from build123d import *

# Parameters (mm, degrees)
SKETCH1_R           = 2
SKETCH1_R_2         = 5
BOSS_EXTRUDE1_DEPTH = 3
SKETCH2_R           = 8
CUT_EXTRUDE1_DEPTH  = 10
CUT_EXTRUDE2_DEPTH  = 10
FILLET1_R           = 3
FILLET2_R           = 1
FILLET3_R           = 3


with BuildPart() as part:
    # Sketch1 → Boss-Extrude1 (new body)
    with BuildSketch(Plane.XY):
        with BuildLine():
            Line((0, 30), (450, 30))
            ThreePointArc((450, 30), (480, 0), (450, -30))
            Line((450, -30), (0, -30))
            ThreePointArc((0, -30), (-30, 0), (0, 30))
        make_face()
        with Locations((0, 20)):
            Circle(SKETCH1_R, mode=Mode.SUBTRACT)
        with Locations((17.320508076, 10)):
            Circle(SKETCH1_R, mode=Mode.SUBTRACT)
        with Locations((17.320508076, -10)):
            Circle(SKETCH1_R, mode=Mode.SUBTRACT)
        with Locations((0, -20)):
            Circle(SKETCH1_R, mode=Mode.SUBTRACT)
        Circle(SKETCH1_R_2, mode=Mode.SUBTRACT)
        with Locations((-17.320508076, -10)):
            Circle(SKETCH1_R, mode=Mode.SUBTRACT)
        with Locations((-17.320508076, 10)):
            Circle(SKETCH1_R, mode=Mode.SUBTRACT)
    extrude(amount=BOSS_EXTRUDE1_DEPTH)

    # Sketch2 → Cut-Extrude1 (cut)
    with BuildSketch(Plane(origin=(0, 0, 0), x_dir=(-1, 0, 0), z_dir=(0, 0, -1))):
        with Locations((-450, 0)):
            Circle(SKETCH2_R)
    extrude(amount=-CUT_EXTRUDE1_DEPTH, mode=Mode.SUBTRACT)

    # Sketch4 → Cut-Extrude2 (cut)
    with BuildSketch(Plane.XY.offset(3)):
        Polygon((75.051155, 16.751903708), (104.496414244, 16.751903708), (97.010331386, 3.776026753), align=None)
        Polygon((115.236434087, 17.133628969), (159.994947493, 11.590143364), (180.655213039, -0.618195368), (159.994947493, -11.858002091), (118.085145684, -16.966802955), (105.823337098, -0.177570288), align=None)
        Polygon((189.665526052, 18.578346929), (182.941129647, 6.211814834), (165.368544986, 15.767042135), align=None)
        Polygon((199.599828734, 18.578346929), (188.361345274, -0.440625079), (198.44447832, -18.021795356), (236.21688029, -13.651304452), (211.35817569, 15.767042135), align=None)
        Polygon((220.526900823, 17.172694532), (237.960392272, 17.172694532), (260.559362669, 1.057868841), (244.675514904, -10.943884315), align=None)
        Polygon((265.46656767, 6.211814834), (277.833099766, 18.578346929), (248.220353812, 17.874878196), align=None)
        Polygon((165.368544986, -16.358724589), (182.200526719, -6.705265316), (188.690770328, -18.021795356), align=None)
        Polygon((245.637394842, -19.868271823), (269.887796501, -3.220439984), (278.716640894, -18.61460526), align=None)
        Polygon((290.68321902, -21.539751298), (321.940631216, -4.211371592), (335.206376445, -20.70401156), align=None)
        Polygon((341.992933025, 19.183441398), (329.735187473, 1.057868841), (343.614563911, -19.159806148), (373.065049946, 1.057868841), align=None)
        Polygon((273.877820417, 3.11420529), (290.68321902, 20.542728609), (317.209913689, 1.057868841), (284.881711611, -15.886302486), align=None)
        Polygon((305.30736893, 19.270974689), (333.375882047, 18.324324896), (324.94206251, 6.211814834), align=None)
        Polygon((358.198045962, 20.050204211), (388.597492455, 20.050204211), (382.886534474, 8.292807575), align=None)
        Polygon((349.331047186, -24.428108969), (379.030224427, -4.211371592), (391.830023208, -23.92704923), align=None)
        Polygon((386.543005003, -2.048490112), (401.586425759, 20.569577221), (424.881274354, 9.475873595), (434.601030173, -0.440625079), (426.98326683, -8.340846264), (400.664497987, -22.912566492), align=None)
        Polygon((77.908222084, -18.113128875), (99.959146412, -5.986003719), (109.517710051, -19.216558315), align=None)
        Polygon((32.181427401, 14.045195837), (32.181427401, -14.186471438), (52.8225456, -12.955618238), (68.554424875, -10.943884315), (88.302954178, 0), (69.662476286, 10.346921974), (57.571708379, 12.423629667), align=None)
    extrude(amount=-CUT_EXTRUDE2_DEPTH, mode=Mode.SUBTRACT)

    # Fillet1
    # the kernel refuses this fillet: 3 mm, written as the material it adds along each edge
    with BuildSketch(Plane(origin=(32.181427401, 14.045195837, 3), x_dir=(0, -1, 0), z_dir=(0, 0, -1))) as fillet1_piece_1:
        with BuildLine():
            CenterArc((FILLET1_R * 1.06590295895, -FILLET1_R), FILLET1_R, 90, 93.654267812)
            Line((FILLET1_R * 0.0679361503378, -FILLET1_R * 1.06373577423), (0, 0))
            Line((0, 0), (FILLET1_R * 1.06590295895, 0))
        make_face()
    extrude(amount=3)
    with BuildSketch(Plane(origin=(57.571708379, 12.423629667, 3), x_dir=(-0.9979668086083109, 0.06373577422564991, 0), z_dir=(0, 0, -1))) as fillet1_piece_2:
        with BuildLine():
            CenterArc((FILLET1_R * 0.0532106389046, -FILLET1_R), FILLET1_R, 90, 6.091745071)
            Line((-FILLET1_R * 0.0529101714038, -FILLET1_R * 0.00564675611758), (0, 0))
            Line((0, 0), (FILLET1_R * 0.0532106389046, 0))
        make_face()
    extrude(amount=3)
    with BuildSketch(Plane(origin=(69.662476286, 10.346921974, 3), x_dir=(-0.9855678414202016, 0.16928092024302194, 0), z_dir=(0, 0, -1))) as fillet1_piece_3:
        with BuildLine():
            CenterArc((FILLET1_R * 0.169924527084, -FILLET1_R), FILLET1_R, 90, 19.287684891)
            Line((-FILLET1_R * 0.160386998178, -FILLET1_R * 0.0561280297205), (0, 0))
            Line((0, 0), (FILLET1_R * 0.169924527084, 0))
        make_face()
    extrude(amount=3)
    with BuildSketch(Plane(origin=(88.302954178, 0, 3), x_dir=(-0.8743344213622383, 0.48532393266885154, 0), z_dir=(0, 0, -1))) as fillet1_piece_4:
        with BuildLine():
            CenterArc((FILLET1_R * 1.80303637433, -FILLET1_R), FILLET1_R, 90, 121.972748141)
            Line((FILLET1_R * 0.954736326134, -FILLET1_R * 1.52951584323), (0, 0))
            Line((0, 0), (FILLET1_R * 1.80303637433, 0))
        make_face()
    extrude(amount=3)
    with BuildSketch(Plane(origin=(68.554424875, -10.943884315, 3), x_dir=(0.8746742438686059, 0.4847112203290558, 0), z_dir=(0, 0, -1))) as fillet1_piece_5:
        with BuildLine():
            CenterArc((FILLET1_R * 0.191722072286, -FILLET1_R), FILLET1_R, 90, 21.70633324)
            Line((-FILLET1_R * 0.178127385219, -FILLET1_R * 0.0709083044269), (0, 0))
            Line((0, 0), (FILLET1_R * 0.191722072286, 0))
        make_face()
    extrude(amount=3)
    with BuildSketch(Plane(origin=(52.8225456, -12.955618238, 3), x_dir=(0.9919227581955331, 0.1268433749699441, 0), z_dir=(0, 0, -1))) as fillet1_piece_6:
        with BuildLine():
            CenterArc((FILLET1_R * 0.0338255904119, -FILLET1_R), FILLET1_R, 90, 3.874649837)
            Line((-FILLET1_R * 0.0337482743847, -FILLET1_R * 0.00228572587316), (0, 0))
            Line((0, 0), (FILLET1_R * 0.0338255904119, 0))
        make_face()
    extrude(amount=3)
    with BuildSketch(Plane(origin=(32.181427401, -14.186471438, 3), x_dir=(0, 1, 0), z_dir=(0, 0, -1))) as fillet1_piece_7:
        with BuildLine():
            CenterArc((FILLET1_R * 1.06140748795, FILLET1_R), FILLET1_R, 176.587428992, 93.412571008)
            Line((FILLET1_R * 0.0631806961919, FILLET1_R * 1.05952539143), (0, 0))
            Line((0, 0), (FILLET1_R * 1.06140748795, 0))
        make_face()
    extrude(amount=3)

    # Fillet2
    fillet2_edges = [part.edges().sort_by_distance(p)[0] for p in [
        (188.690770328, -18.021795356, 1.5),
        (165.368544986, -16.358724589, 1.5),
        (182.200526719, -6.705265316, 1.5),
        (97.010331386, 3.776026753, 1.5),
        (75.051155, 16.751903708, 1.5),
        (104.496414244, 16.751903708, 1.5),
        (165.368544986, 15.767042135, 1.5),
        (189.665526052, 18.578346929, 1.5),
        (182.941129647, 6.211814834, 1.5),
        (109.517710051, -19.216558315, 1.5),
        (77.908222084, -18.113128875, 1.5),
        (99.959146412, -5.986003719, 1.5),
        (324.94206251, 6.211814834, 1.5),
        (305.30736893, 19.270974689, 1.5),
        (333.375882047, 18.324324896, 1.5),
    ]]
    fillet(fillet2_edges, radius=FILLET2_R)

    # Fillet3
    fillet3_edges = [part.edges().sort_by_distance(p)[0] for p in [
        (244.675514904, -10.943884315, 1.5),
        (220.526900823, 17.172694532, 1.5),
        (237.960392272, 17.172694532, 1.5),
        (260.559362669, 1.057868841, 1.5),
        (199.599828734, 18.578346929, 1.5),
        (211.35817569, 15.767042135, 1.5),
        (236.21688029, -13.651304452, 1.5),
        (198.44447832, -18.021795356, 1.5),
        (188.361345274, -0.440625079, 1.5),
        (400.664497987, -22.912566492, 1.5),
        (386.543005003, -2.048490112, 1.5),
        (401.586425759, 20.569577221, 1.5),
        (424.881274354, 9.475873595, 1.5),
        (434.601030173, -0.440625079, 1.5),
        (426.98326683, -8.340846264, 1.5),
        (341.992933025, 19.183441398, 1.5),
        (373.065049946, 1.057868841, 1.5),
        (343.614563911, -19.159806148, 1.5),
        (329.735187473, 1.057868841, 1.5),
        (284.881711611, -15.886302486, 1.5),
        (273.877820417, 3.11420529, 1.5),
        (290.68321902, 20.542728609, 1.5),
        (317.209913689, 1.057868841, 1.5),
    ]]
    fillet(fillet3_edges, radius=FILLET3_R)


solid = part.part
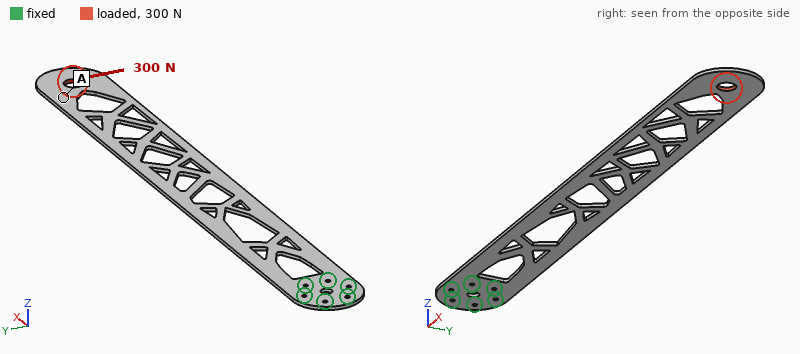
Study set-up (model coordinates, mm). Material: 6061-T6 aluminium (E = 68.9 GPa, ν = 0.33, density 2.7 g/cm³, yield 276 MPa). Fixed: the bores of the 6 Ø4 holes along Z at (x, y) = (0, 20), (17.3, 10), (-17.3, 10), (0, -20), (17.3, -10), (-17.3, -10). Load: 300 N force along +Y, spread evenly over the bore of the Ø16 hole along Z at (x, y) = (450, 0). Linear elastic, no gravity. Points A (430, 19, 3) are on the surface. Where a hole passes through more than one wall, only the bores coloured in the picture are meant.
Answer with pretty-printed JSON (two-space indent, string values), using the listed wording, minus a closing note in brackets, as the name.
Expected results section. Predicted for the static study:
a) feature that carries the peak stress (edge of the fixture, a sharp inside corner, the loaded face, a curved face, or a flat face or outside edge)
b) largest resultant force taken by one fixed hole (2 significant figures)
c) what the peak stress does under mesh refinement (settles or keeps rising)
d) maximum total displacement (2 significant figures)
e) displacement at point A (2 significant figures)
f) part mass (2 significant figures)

{
  "feature that carries the peak stress": "edge of the fixture",
  "largest resultant force taken by one fixed hole": "1.6 kN",
  "what the peak stress does under mesh refinement": "keeps rising",
  "maximum total displacement": "3.2 mm",
  "displacement at point A": "2.7 mm",
  "part mass": "160 g"
}
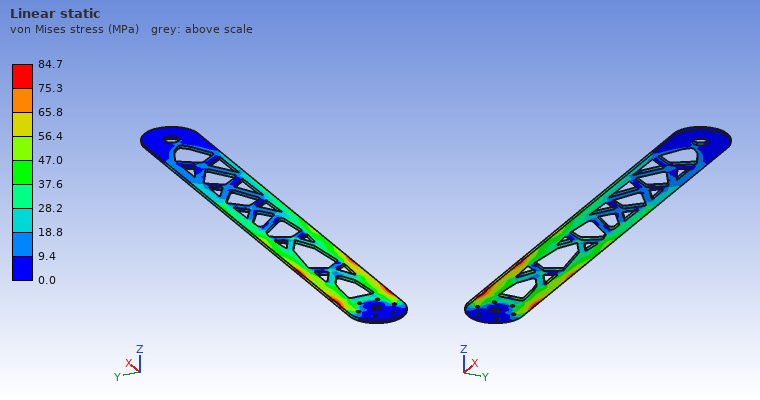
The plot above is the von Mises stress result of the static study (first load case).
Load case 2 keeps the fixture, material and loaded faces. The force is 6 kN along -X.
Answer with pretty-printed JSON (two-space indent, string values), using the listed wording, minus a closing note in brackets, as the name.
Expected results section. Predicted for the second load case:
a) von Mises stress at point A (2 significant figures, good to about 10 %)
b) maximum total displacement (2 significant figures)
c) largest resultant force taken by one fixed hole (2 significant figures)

{
  "von Mises stress at point A": "50 MPa",
  "maximum total displacement": "0.55 mm",
  "largest resultant force taken by one fixed hole": "1.5 kN"
}
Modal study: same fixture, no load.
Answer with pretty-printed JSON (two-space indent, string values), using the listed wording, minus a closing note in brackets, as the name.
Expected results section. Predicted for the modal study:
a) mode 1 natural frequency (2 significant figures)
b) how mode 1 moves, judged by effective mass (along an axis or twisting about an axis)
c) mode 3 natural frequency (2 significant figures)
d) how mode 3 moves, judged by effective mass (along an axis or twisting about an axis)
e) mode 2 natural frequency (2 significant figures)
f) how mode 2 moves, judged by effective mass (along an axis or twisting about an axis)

{
  "mode 1 natural frequency": "11 Hz",
  "how mode 1 moves, judged by effective mass": "along Z",
  "mode 3 natural frequency": "140 Hz",
  "how mode 3 moves, judged by effective mass": "twisting about X",
  "mode 2 natural frequency": "66 Hz",
  "how mode 2 moves, judged by effective mass": "along Z"
}
